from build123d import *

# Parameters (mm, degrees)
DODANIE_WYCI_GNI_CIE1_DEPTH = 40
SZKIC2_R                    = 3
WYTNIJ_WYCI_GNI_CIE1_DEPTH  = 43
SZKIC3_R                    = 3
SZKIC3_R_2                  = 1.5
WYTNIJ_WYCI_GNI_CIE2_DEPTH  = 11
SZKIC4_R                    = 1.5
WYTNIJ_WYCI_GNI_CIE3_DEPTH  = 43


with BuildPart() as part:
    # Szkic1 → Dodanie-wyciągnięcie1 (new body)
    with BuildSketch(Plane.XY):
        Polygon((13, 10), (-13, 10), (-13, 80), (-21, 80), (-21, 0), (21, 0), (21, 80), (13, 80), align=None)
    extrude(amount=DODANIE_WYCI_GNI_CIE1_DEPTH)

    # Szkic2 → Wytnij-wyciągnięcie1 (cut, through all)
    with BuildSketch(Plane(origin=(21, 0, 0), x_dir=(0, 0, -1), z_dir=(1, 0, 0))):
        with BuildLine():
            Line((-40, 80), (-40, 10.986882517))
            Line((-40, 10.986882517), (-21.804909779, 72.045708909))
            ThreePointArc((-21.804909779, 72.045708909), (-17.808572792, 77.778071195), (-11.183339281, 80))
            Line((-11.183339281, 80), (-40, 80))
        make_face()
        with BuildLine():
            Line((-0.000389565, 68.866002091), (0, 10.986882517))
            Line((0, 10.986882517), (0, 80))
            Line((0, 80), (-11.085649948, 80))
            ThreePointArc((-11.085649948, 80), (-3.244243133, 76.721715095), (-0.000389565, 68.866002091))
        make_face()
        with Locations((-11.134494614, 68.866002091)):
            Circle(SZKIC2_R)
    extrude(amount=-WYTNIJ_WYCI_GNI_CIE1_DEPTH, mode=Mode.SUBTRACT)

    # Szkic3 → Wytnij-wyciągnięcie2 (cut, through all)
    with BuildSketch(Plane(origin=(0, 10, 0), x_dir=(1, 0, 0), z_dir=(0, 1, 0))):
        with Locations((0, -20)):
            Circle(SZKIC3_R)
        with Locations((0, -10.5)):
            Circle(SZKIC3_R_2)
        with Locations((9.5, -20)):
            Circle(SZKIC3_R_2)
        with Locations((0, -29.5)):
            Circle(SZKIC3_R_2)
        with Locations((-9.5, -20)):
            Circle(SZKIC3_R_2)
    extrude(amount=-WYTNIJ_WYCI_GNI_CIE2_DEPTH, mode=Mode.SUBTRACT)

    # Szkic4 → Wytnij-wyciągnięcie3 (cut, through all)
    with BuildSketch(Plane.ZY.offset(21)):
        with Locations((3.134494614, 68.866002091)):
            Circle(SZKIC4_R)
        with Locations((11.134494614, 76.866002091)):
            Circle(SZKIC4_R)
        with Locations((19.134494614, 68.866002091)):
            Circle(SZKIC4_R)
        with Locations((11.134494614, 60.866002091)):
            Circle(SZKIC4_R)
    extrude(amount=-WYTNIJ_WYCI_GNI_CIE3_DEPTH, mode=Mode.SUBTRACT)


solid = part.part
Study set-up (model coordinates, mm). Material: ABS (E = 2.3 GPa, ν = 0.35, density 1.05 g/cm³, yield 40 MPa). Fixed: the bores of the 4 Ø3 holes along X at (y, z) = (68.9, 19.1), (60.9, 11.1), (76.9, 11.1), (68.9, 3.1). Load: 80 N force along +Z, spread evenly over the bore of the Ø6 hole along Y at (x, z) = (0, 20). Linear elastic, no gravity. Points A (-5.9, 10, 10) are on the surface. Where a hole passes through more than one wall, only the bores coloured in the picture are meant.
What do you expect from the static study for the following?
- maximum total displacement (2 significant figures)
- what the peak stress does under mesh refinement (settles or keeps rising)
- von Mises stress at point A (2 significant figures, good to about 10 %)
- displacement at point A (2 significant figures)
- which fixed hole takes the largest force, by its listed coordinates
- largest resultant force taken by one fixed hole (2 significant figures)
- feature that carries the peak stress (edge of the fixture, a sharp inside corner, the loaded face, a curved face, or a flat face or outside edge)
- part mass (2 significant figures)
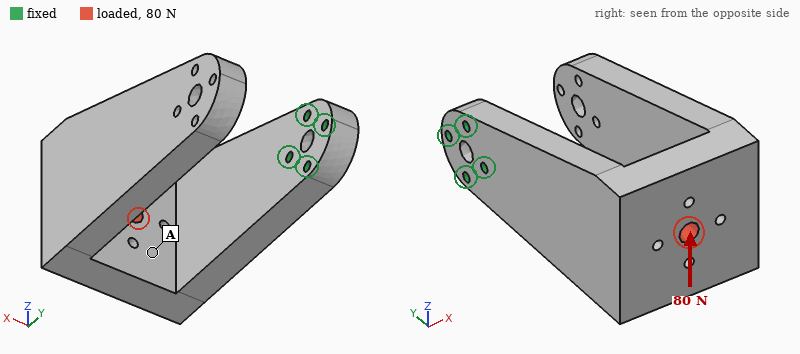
1.1 mm
keeps rising
1.1 MPa
0.44 mm
(68.9, 19.1)
240 N
edge of the fixture
51 g
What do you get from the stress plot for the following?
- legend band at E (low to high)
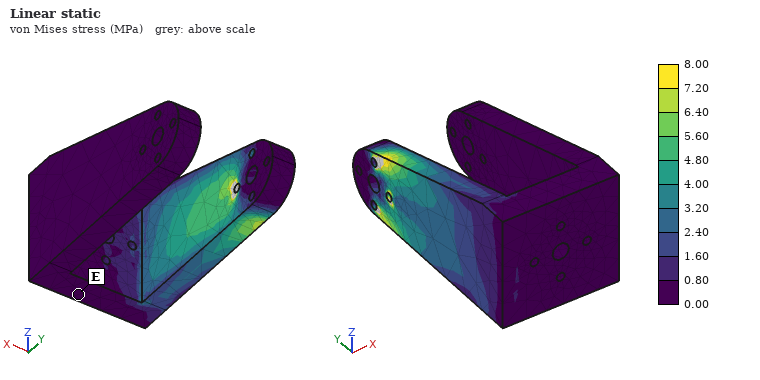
0.00 to 0.80 MPa
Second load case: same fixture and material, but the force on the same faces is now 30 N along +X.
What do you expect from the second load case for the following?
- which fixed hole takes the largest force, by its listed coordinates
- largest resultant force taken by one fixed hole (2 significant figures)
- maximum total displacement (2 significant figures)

(60.9, 11.1)
98 N
1.1 mm
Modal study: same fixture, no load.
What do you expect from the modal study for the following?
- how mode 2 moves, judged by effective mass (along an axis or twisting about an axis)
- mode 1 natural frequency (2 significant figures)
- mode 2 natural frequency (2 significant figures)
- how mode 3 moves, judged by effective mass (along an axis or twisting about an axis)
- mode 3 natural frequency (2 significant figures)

along Z
160 Hz
220 Hz
along X
280 Hz
